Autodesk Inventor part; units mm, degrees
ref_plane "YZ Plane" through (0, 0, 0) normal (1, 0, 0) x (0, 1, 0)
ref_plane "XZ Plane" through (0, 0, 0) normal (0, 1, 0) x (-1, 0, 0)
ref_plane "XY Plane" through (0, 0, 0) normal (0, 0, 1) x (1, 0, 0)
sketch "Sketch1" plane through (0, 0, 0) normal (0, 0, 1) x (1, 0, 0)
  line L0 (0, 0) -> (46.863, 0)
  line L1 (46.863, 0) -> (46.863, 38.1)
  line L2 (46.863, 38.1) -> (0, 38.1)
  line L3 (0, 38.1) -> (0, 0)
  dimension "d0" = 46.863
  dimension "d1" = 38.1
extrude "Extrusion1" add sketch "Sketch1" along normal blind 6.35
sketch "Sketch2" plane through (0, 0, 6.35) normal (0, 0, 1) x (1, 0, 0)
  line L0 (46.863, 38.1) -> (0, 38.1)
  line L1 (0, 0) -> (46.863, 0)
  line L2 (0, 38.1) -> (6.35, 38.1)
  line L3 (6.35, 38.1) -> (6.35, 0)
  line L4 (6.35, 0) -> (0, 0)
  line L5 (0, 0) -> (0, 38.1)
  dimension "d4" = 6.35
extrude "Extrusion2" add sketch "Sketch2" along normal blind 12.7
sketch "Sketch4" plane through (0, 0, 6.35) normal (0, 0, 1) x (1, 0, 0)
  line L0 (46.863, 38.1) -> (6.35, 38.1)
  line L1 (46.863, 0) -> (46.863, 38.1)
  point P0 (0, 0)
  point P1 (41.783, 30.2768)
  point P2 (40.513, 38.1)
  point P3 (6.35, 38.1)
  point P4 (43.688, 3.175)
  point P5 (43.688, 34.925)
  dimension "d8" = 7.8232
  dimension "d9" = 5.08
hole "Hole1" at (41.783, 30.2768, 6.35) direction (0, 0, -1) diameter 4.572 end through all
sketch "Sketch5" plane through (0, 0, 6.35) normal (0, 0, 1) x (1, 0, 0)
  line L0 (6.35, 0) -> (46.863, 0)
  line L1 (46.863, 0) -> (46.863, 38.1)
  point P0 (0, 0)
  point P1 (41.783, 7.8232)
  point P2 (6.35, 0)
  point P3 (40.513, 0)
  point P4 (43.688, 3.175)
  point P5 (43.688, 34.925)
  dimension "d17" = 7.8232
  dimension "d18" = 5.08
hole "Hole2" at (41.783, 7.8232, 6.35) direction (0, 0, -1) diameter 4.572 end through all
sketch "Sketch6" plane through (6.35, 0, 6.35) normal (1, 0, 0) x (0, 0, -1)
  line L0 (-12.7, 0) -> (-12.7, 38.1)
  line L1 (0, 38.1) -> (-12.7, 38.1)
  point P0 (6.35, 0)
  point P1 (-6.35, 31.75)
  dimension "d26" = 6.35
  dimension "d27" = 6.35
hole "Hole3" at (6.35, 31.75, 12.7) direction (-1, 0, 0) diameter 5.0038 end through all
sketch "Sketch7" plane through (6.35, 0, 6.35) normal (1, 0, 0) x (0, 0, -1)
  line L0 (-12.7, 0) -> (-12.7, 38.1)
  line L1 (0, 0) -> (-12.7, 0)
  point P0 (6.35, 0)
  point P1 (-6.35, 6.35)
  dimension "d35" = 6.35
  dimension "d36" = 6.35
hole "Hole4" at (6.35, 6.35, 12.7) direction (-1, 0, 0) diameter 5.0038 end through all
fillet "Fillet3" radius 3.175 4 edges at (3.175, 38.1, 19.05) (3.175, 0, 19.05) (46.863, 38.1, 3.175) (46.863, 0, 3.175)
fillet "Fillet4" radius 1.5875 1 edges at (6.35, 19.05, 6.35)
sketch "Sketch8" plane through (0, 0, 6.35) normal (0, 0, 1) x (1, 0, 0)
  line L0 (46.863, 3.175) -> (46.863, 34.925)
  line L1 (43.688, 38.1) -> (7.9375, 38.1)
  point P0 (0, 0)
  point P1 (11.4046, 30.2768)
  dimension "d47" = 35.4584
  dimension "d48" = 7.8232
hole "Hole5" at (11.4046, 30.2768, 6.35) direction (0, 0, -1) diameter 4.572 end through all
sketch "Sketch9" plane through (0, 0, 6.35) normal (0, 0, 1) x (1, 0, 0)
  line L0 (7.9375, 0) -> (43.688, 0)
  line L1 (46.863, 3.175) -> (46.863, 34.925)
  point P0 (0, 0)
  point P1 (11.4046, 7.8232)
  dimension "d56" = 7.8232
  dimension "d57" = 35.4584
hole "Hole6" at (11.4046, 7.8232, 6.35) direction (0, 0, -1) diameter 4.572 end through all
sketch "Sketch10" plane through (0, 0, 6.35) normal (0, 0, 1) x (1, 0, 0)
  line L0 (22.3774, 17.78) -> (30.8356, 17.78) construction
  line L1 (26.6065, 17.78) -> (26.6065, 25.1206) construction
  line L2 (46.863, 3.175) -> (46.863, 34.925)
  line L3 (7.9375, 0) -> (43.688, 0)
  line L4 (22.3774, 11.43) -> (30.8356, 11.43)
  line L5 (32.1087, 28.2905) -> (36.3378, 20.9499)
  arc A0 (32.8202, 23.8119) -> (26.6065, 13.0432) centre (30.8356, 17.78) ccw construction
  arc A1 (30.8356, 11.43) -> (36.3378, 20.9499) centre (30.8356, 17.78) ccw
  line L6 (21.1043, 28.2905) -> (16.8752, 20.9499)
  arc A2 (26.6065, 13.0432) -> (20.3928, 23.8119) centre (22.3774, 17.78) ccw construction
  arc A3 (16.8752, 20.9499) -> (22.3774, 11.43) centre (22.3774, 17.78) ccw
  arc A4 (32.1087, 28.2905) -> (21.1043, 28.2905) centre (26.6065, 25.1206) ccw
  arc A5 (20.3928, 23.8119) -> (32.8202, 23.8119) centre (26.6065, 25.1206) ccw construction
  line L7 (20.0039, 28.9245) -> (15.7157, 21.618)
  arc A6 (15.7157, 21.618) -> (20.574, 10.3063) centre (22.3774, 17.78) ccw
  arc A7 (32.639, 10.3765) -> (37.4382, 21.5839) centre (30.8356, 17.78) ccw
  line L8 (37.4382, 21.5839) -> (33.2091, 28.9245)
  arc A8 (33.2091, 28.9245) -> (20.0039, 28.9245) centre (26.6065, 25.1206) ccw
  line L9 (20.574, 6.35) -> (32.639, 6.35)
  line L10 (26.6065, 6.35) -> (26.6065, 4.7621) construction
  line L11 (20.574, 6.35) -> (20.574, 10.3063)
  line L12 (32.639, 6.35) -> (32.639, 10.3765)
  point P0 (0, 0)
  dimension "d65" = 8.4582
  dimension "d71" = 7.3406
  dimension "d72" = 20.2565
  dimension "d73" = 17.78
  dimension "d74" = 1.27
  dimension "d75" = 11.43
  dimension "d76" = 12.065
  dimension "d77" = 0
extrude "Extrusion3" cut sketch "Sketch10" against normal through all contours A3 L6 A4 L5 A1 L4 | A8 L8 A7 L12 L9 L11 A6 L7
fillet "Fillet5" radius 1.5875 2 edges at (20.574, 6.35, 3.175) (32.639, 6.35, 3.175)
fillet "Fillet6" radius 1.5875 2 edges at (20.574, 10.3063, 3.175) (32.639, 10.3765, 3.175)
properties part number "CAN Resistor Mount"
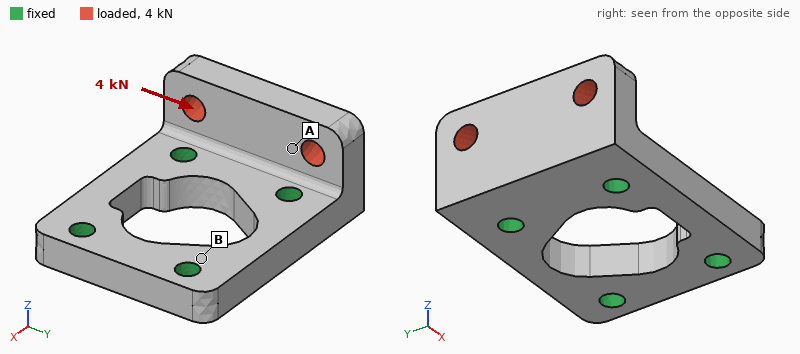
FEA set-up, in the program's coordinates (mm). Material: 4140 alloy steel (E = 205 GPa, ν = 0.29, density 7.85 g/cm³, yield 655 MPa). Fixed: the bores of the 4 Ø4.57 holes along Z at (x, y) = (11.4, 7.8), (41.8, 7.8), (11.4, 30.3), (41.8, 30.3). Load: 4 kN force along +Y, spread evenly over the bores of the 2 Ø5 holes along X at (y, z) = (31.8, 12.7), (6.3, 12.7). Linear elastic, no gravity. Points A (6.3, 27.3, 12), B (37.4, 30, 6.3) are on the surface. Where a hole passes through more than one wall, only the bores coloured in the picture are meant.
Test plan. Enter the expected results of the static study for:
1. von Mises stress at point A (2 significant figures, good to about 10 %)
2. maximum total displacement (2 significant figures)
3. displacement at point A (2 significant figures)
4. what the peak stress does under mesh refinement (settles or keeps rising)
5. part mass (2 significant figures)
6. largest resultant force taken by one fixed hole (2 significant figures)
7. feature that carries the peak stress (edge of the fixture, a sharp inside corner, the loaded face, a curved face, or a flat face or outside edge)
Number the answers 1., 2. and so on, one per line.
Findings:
1. 44 MPa
2. 9.9 µm
3. 5.9 µm
4. keeps rising
5. 85 g
6. 2.7 kN
7. edge of the fixture
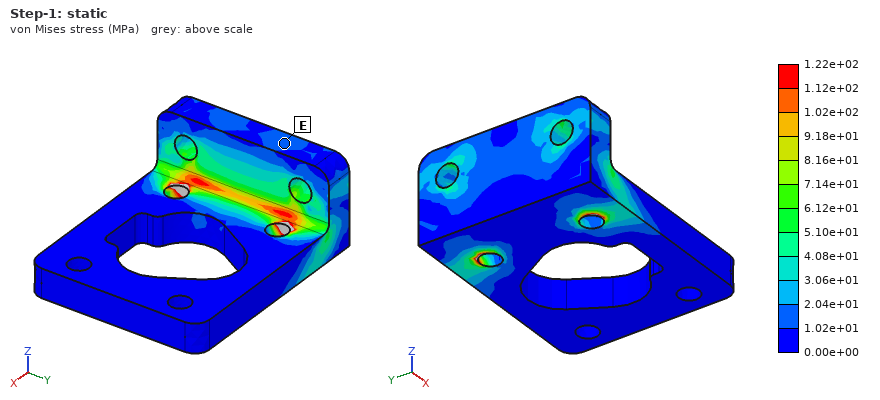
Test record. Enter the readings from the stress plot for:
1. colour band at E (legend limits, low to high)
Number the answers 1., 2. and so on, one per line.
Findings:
1. 1.02e+01 to 2.04e+01 MPa
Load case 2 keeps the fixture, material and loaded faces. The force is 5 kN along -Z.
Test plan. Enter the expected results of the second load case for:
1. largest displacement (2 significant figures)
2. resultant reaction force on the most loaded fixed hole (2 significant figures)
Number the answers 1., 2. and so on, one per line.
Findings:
1. 22 µm
2. 2.6 kN
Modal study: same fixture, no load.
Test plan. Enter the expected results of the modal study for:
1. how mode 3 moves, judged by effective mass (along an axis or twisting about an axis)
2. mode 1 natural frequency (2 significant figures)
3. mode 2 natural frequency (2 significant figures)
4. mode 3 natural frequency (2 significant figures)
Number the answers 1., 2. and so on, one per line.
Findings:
1. along Y
2. 12 kHz
3. 19 kHz
4. 27 kHz
